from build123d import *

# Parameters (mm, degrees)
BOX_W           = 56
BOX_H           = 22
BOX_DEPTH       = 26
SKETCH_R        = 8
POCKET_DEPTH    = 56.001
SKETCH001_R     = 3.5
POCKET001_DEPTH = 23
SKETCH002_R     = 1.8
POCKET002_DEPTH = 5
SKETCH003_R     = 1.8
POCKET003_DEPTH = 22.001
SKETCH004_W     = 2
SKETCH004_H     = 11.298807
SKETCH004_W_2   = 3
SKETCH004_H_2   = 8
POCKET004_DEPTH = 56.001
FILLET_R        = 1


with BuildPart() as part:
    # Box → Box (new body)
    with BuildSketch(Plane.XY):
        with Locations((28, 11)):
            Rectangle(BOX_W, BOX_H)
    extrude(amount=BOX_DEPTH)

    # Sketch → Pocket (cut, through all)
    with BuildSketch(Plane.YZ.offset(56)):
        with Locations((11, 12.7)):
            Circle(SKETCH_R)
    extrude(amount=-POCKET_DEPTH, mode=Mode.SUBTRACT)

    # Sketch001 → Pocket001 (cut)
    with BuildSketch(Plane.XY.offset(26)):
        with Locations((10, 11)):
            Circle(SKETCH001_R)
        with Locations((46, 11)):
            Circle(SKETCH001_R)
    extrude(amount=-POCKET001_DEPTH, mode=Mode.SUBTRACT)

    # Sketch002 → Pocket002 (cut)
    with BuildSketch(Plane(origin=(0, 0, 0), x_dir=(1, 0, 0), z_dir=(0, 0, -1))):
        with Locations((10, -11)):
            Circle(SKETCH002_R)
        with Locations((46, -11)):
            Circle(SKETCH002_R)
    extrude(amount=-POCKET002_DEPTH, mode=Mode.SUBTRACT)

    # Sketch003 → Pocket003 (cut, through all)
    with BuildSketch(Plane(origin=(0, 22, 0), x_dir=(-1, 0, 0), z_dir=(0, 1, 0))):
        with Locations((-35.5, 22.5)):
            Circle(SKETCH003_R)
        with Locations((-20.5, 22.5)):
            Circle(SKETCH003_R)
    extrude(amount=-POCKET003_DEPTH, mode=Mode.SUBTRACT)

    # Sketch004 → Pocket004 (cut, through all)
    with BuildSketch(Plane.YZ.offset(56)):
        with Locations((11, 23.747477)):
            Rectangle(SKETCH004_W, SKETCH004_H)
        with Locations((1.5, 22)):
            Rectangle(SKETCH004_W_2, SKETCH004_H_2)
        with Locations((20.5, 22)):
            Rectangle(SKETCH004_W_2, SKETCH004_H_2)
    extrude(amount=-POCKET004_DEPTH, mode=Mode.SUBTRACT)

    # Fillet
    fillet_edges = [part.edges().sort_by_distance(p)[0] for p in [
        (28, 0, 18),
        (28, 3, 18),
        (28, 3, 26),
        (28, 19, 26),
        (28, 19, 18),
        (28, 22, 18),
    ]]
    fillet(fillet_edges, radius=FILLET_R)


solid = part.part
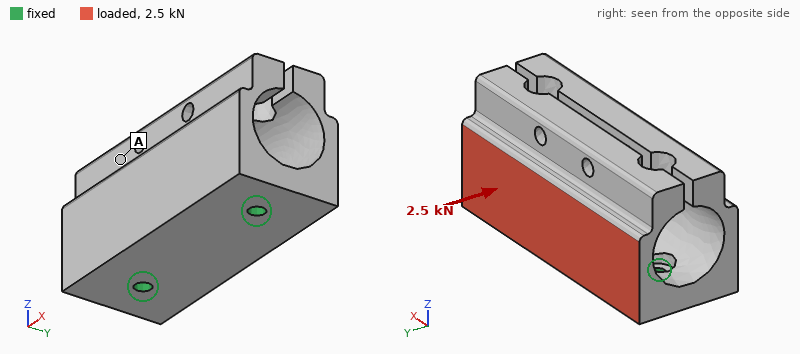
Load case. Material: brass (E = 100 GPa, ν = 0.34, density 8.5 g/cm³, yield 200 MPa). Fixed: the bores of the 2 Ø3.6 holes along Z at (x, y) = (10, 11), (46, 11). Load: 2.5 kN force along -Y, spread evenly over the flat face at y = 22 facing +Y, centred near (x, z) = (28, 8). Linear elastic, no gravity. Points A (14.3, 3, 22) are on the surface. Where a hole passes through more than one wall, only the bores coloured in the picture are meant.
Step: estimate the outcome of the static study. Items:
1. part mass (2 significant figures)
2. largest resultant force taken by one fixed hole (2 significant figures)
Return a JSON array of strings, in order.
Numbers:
["140 g", "1.3 kN"]
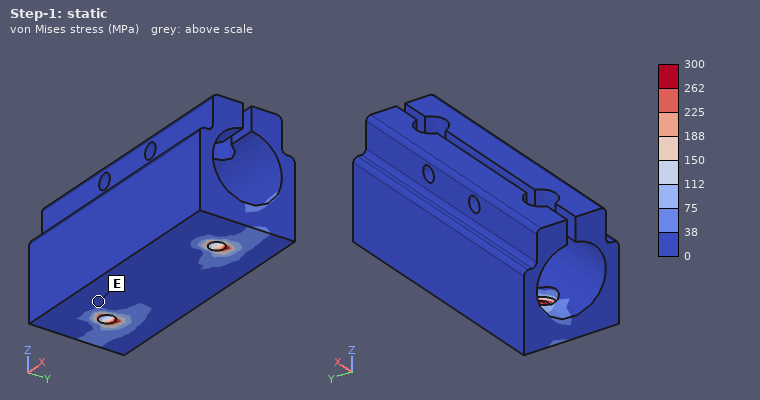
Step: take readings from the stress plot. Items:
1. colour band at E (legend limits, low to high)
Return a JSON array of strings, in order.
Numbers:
["0 to 38 MPa"]
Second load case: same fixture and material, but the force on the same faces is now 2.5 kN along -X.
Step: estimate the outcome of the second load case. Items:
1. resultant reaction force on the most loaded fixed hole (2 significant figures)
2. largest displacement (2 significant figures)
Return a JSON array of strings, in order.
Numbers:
["1.5 kN", "12 µm"]
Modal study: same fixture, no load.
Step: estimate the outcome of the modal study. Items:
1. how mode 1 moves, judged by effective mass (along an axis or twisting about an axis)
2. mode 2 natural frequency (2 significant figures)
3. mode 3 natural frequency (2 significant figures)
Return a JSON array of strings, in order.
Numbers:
["along Y", "2900 Hz", "3600 Hz"]
